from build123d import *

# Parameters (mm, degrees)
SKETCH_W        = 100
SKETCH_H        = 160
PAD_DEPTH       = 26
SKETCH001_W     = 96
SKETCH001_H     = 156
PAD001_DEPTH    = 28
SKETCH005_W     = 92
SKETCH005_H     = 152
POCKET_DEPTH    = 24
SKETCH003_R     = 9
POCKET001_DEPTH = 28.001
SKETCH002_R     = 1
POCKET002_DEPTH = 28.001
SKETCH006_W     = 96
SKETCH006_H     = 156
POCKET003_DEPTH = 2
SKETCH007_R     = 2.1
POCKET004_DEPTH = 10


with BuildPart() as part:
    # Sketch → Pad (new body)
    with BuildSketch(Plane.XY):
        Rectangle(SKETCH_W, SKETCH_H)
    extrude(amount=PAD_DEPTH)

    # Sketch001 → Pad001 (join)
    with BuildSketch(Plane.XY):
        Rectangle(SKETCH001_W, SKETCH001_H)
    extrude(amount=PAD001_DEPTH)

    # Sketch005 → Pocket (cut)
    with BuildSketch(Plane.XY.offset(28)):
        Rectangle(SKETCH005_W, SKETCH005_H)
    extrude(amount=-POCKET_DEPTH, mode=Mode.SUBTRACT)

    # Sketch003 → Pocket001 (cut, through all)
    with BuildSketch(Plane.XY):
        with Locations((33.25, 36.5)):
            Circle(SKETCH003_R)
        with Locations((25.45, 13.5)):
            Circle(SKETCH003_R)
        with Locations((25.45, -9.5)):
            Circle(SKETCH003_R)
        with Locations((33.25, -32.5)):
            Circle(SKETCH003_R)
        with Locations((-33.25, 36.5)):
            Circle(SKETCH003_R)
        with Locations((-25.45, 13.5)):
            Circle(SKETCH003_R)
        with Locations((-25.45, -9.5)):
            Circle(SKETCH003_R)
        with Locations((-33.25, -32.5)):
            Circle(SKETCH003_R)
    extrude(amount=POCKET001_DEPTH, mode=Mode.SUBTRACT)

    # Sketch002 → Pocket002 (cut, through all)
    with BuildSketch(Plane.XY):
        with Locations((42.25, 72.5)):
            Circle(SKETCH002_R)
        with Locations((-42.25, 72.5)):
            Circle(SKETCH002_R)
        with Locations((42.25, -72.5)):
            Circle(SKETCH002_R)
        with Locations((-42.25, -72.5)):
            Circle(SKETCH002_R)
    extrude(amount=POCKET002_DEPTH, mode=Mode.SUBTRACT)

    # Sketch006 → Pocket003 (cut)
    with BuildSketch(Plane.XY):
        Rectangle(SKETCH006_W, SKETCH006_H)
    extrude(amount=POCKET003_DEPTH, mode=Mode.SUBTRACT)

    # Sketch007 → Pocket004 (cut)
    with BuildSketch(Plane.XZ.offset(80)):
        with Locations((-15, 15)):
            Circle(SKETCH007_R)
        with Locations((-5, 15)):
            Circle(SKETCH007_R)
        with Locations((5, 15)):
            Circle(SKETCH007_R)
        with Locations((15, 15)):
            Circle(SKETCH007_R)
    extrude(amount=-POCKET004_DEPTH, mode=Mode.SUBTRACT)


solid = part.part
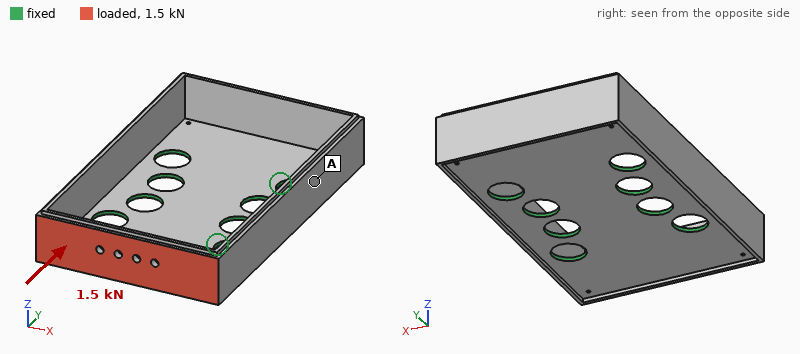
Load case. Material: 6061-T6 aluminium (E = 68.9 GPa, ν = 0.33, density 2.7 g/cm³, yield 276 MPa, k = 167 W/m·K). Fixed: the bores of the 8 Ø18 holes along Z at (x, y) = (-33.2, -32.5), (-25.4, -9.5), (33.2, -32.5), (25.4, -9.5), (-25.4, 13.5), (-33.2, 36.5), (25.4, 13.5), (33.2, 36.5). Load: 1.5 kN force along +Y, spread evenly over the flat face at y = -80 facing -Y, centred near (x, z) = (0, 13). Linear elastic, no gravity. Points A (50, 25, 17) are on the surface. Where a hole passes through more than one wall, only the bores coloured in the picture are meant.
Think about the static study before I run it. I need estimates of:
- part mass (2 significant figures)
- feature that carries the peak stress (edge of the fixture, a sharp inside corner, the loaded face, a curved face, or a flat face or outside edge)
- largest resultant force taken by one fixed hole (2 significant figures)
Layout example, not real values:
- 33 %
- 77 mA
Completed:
- 210 g
- a flat face or outside edge
- 440 N
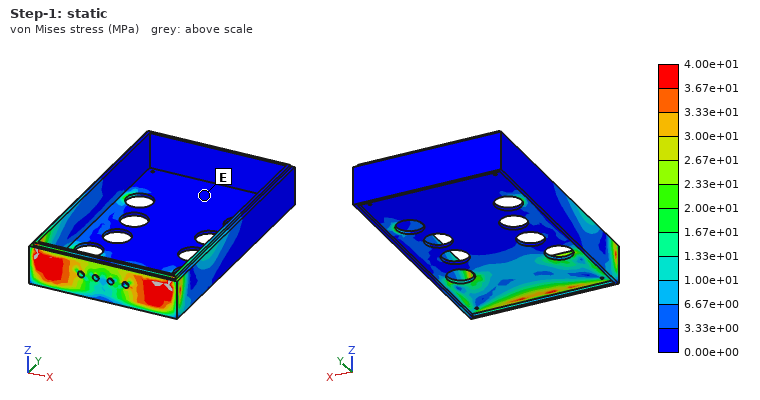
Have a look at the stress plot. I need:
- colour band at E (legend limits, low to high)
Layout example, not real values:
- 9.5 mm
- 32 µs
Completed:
- 0.00e+00 to 3.33e+00 MPa
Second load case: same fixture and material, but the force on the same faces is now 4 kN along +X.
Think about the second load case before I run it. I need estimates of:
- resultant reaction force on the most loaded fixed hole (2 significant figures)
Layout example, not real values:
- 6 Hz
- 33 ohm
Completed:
- 3.2 kN
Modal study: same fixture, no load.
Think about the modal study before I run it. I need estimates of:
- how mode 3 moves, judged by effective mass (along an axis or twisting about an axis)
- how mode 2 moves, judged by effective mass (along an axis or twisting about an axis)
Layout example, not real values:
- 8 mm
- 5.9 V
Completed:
- along Z
- along X
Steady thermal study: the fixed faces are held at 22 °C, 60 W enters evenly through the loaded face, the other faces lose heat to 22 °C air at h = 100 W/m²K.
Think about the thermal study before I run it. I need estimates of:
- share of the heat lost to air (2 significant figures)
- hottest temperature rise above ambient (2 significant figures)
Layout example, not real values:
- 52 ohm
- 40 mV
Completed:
- 52 %
- 36 K
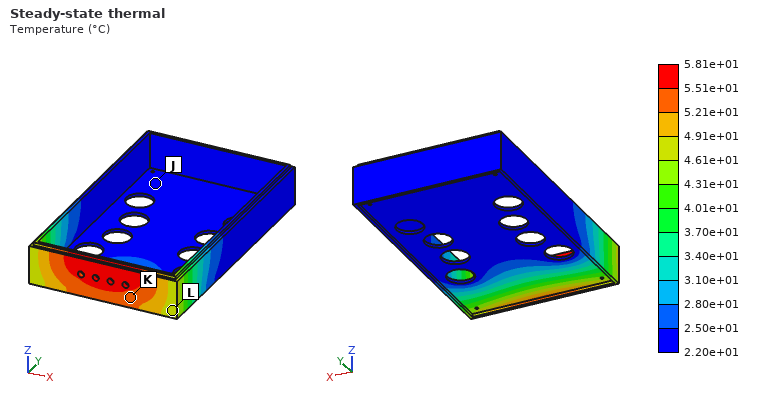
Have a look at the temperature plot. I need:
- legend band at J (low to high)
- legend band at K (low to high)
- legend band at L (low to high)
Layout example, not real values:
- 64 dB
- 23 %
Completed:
- 2.20e+01 to 2.50e+01 °C
- 5.21e+01 to 5.51e+01 °C
- 4.61e+01 to 4.91e+01 °C
